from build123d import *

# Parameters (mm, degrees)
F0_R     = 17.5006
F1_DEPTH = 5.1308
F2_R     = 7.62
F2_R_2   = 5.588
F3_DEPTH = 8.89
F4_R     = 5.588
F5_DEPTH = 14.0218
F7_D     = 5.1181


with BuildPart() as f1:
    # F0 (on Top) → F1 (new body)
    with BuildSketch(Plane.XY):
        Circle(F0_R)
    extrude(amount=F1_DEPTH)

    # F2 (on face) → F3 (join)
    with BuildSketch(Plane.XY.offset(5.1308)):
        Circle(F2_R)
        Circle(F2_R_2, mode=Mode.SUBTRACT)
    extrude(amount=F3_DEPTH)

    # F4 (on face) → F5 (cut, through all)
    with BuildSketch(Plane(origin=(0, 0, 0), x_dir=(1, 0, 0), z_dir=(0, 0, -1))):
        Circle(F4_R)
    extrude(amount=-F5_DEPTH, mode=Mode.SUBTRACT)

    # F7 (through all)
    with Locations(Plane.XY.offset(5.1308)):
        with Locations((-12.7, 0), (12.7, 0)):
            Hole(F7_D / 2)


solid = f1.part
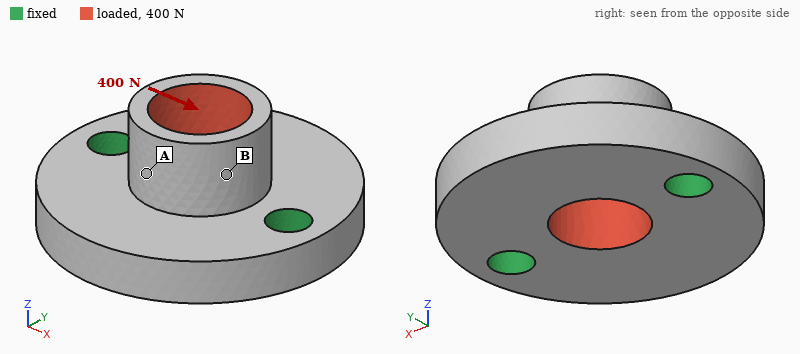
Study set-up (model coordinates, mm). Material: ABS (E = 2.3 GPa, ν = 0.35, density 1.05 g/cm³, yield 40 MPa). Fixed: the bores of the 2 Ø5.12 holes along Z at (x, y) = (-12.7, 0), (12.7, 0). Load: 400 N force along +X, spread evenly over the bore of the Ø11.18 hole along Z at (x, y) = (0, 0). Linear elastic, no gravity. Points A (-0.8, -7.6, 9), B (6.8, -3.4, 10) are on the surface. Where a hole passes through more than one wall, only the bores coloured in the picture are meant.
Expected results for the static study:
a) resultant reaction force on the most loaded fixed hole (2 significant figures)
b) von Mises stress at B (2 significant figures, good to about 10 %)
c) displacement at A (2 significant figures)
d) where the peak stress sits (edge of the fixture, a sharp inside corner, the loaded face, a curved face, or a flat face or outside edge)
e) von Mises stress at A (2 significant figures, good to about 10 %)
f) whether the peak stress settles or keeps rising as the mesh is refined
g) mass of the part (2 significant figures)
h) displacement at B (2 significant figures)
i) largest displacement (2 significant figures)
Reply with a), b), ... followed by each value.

a) 220 N
b) 2.0 MPa
c) 38 µm
d) edge of the fixture
e) 4.4 MPa
f) keeps rising
g) 5.2 g
h) 50 µm
i) 71 µm
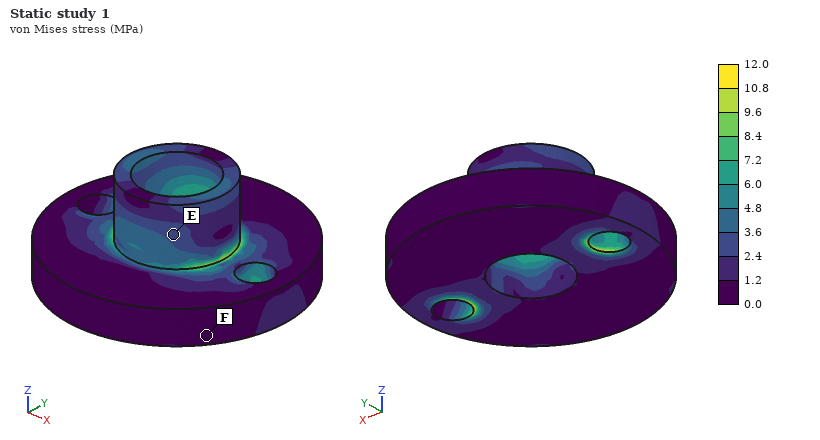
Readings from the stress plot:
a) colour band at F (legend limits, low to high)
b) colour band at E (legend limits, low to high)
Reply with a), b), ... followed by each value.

a) 0.0 to 1.2 MPa
b) 2.4 to 3.6 MPa
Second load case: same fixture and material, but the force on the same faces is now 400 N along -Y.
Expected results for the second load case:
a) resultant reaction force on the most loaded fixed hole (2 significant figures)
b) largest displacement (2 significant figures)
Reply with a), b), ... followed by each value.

a) 200 N
b) 0.16 mm
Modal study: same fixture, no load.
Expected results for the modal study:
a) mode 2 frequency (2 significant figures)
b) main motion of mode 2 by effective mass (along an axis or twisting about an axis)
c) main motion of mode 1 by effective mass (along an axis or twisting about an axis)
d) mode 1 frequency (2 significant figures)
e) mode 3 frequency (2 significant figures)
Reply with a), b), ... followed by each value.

a) 5100 Hz
b) along Z
c) twisting about X
d) 4000 Hz
e) 10000 Hz
